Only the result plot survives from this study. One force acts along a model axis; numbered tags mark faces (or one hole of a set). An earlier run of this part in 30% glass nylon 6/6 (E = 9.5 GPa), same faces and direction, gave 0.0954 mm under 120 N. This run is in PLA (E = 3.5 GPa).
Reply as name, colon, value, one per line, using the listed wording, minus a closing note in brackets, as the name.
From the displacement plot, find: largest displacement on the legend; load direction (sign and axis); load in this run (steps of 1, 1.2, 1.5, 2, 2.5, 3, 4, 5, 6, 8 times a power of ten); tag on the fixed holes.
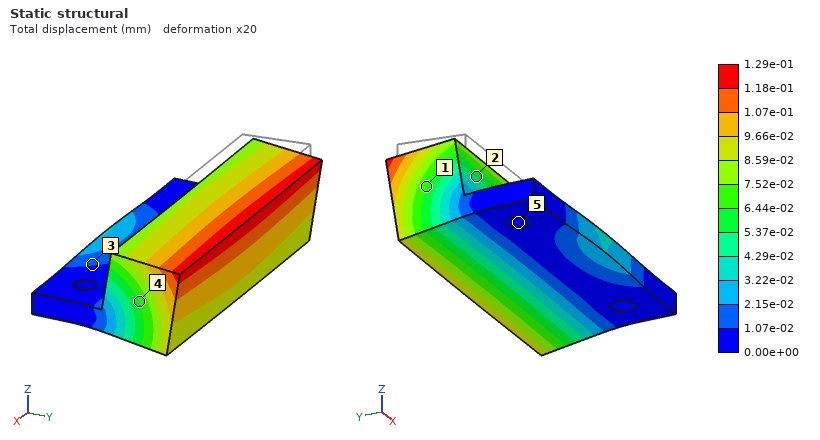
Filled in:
largest displacement on the legend: 1.29e-01 mm
load direction: +Y
load in this run: 60 N
tag on the fixed holes: 5
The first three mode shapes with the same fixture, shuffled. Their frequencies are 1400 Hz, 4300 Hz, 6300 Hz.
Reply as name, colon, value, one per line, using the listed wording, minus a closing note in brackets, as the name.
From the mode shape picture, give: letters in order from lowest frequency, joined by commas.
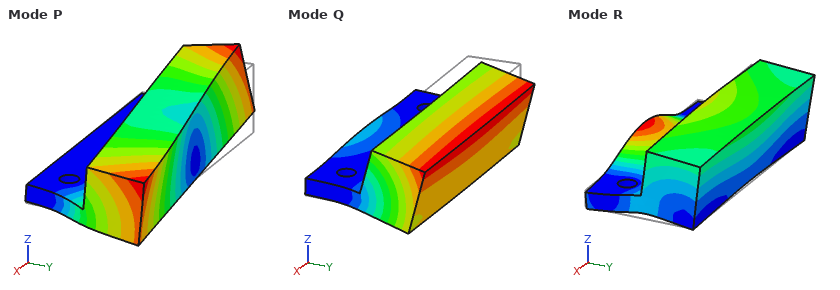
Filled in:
letters in order from lowest frequency, joined by commas: Q, P, R
